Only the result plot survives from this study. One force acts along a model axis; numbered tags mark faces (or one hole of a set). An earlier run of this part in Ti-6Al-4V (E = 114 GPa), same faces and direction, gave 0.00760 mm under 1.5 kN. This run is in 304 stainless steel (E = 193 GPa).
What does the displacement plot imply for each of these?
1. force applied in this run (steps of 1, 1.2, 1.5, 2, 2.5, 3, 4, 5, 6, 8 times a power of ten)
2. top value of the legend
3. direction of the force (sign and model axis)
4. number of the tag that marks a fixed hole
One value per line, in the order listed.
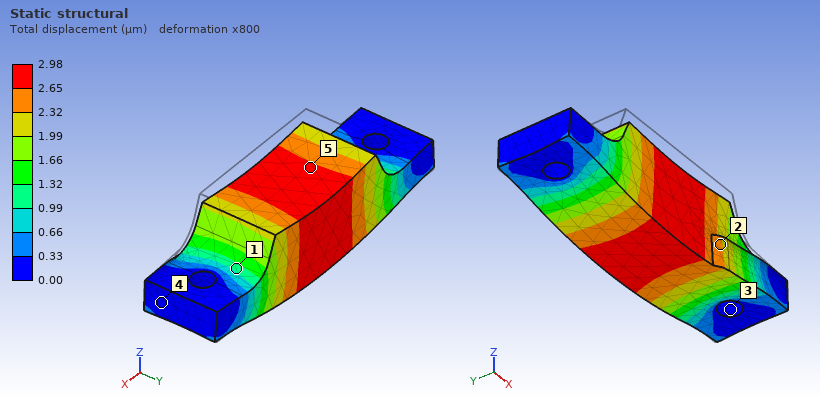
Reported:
1 kN
2.98 µm
-Z
3
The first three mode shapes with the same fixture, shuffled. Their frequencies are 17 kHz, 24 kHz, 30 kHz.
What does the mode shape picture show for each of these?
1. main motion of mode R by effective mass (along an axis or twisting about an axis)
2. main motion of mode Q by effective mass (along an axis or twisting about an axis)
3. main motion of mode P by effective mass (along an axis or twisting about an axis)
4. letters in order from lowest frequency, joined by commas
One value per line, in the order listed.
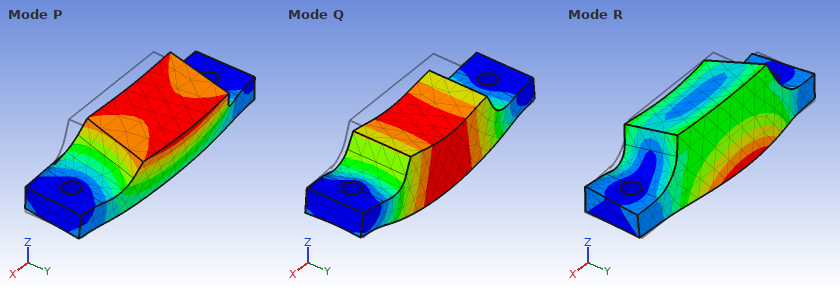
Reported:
along Y
along Z
along Y
P, Q, R
